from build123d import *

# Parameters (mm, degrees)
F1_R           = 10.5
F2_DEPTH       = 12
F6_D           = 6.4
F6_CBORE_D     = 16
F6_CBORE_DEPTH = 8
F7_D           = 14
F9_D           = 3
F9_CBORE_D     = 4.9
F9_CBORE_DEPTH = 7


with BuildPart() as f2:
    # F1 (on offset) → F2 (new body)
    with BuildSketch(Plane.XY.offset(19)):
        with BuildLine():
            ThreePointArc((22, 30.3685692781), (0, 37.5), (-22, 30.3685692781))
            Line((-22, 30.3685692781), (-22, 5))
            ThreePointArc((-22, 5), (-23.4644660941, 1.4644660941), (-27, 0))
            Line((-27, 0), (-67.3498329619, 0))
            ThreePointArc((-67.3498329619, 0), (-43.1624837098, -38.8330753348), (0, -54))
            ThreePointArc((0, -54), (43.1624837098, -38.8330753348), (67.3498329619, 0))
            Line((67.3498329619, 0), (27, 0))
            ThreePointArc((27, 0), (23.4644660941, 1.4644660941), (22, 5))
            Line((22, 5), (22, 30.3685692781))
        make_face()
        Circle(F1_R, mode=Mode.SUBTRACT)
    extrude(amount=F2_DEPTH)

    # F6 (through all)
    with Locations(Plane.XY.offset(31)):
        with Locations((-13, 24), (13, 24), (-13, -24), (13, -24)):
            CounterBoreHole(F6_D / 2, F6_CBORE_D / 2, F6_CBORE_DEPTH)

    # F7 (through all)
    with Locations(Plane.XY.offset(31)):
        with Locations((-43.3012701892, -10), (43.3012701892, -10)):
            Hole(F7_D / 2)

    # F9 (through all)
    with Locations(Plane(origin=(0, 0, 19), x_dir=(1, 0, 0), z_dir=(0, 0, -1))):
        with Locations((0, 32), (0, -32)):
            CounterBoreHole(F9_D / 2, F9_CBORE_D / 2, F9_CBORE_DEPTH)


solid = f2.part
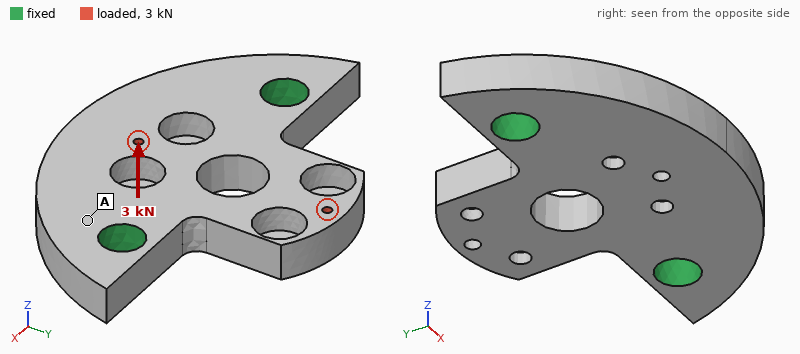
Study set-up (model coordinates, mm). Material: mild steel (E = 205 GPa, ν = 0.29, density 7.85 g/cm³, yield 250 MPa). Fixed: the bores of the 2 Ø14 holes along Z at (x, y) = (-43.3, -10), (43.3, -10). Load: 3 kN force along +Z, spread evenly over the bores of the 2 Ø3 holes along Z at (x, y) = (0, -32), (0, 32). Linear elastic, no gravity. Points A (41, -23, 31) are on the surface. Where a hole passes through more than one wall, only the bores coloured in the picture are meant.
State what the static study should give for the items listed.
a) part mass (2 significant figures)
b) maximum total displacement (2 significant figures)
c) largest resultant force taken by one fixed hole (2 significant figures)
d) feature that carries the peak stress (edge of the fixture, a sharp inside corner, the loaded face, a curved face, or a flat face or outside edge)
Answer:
540 g
87 µm
1.5 kN
the loaded face
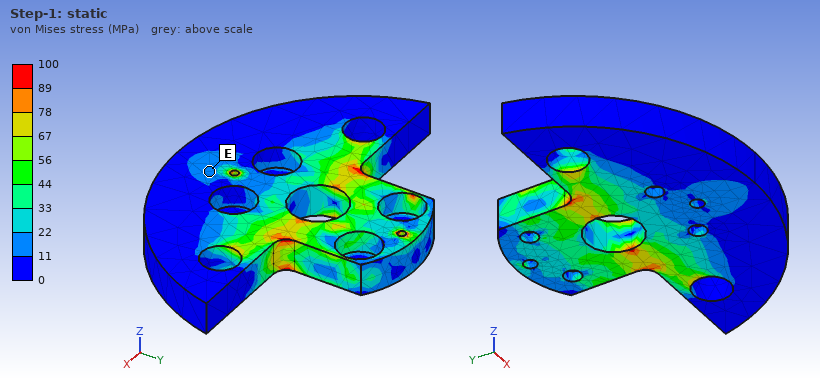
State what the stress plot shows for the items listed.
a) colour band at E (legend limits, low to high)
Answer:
11 to 22 MPa
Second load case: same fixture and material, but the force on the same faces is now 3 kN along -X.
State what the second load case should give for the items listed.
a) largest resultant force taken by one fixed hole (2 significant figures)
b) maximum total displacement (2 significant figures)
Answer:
1.6 kN
11 µm
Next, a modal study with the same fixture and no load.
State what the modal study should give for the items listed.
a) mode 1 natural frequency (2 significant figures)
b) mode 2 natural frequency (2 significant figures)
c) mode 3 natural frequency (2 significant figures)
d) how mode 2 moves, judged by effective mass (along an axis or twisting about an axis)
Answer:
3300 Hz
5000 Hz
9600 Hz
along Z
